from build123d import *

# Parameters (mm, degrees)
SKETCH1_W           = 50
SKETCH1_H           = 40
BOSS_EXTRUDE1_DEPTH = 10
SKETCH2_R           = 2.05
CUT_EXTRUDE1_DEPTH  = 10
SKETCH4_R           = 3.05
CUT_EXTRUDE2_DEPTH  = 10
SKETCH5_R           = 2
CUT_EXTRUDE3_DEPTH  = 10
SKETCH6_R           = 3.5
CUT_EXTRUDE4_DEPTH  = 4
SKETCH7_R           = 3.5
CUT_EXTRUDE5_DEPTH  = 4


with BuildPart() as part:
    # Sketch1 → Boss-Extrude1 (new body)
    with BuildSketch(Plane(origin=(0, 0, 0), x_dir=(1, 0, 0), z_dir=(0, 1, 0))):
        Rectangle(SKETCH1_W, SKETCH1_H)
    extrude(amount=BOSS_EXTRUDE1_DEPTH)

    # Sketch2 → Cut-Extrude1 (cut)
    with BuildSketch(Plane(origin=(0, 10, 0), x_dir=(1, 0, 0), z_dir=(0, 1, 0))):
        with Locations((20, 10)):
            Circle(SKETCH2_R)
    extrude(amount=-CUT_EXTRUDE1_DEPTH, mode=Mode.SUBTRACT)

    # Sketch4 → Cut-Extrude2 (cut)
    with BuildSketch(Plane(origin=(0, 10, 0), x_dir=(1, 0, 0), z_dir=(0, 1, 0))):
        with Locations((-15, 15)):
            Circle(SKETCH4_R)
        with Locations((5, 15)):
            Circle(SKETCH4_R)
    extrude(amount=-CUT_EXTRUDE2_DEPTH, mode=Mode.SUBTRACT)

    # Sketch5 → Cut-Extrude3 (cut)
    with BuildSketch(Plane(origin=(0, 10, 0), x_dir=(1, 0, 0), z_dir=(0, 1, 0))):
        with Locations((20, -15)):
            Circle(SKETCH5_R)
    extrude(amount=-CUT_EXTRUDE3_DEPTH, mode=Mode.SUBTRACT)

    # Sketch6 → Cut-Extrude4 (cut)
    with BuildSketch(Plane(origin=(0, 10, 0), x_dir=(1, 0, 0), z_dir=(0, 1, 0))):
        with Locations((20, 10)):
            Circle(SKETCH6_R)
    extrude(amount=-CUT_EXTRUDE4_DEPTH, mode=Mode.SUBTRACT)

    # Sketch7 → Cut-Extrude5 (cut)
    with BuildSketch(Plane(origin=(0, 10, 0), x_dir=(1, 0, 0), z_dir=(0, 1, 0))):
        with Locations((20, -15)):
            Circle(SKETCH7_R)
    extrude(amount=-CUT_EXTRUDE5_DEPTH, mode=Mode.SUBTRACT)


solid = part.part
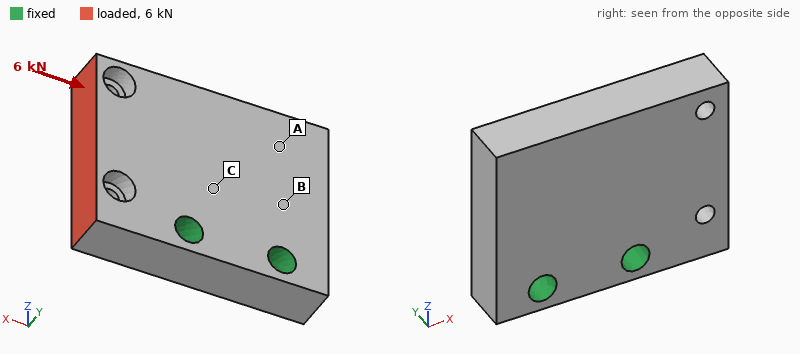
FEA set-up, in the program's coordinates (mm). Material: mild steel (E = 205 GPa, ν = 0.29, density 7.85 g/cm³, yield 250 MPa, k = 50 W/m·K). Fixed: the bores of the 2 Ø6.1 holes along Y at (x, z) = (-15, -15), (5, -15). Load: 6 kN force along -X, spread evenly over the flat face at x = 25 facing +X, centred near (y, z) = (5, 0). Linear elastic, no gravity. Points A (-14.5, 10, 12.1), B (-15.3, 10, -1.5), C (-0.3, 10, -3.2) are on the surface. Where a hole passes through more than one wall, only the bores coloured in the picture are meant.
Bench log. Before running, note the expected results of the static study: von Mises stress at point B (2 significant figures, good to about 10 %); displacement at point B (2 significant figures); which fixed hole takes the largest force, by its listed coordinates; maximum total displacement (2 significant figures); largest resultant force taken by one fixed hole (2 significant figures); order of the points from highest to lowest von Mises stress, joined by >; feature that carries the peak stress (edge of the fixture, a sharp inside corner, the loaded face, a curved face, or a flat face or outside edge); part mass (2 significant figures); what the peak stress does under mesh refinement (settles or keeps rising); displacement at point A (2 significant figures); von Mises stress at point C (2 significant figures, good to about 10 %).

17 MPa
2.9 µm
(5, -15)
13 µm
5.2 kN
C > B > A
edge of the fixture
150 g
keeps rising
5.9 µm
29 MPa
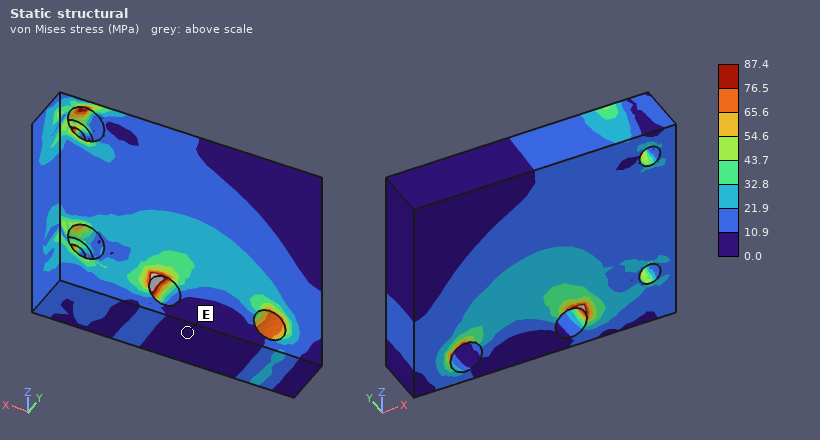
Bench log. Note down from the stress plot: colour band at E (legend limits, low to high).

0.0 to 10.9 MPa
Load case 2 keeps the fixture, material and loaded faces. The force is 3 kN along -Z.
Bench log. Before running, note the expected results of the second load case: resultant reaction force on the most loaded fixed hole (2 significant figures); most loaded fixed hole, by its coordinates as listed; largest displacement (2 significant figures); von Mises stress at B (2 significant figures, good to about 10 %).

5.0 kN
(5, -15)
11 µm
11 MPa
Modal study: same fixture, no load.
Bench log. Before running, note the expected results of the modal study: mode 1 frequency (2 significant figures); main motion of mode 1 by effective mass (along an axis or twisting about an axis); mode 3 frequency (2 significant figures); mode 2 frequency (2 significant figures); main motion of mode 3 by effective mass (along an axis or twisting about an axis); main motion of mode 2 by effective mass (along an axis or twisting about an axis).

6000 Hz
along Y
12 kHz
9800 Hz
along X
twisting about Z
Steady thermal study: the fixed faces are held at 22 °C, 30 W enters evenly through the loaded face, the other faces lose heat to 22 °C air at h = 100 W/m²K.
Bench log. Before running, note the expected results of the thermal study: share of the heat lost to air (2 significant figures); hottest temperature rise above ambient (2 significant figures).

25 %
47 K
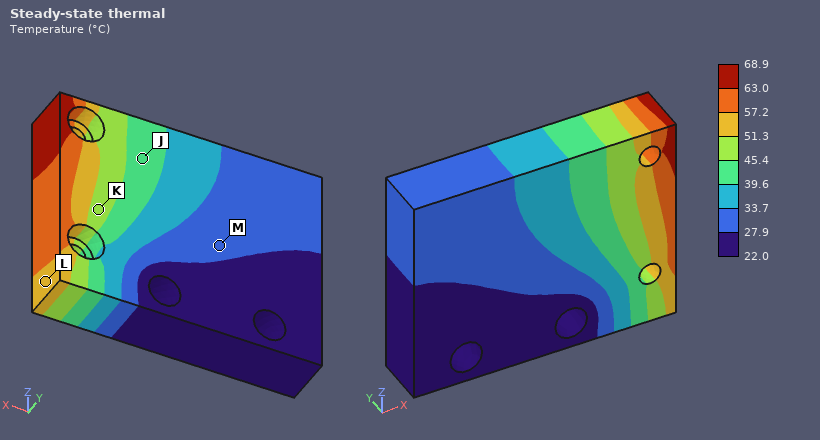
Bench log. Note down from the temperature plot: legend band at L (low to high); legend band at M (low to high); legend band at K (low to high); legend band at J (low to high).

51.3 to 57.2 °C
27.9 to 33.7 °C
45.4 to 51.3 °C
39.6 to 45.4 °C
